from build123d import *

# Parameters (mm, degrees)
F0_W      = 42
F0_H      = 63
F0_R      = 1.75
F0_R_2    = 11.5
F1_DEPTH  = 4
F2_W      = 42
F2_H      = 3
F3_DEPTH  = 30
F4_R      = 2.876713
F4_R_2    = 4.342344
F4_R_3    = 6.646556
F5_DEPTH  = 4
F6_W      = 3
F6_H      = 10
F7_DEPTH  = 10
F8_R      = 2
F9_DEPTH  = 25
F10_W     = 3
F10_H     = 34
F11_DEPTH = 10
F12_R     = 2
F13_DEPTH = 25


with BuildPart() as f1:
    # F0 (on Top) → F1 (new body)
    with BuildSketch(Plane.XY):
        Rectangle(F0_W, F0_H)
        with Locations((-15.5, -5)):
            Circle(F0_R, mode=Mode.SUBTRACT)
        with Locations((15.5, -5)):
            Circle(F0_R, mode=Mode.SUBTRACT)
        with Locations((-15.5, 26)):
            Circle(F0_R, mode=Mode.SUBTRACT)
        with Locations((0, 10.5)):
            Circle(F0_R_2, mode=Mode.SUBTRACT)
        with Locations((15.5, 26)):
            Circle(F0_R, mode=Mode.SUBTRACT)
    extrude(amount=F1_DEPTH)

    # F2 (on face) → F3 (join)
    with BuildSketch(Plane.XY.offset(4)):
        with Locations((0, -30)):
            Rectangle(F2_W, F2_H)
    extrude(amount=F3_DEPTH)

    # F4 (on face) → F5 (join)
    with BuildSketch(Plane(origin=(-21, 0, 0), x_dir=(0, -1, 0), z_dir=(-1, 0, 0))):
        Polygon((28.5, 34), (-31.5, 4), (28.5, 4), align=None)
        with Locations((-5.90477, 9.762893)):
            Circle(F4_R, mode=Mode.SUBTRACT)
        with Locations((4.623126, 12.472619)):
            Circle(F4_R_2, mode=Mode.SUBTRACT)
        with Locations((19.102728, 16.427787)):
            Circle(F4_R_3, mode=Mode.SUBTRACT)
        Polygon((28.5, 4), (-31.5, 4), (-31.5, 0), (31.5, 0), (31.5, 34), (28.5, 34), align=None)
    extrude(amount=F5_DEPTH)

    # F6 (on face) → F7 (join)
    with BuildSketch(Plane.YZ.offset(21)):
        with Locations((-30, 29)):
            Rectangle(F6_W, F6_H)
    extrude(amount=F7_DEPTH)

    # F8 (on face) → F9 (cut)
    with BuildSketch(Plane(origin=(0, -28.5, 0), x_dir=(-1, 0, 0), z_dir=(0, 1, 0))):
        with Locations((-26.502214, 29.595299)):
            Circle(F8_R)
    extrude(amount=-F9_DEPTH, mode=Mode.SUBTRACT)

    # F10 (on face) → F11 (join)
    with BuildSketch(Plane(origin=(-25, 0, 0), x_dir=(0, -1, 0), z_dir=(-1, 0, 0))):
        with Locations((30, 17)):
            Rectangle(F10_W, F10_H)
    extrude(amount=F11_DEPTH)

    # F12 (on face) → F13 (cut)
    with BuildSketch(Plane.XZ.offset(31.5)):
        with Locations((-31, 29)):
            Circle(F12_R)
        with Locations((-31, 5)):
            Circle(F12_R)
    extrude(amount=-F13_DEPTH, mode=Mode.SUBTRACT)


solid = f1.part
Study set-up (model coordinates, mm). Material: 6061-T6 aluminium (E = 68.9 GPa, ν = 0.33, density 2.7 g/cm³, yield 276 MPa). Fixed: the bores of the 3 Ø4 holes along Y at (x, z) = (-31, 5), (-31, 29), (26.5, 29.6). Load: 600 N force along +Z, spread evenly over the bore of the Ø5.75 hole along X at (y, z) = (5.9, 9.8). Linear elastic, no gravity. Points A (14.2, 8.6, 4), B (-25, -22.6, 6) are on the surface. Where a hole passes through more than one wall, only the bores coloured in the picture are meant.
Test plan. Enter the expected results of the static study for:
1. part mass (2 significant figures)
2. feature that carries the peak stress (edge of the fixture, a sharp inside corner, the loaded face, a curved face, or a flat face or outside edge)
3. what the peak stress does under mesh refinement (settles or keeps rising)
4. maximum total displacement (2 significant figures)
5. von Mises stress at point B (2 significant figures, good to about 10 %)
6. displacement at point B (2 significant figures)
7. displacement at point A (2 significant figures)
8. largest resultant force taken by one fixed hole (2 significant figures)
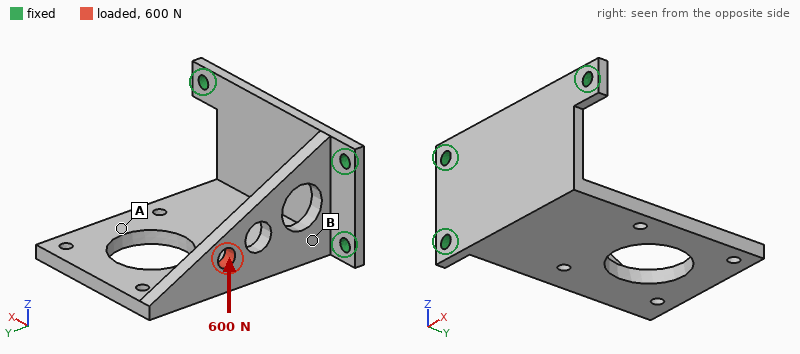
48 g
edge of the fixture
keeps rising
0.19 mm
29 MPa
0.029 mm
0.12 mm
930 N
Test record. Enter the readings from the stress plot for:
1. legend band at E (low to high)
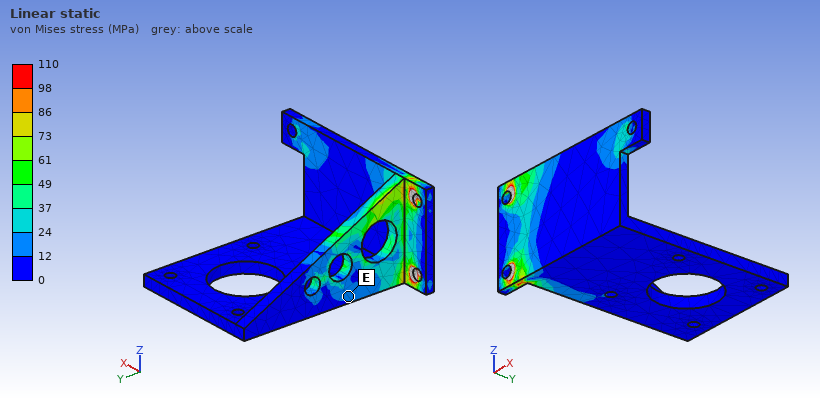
12 to 24 MPa
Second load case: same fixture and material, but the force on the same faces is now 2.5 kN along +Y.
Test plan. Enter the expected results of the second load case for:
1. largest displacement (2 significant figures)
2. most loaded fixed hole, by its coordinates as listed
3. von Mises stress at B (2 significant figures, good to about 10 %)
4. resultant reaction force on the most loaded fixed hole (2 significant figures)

0.32 mm
(-31, 5)
66 MPa
1.9 kN
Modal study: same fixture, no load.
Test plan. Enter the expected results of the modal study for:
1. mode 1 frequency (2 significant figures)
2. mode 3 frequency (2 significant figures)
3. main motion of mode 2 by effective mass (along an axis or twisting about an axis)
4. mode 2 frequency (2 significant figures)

920 Hz
3400 Hz
along Z
1500 Hz
